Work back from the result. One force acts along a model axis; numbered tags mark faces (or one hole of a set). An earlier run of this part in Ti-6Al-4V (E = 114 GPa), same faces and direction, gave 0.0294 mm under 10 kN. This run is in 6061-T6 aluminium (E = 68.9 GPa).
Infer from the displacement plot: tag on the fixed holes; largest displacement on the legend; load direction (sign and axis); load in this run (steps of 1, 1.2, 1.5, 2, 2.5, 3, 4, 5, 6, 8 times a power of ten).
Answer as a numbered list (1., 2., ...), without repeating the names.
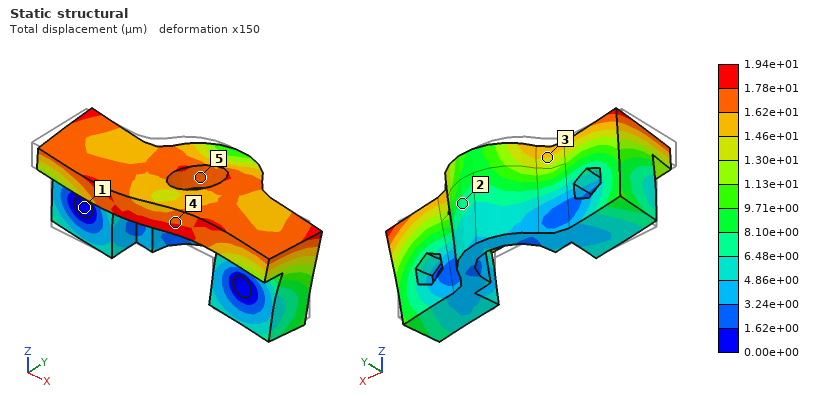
1. 1
2. 1.94e+01 µm
3. +X
4. 4 kN
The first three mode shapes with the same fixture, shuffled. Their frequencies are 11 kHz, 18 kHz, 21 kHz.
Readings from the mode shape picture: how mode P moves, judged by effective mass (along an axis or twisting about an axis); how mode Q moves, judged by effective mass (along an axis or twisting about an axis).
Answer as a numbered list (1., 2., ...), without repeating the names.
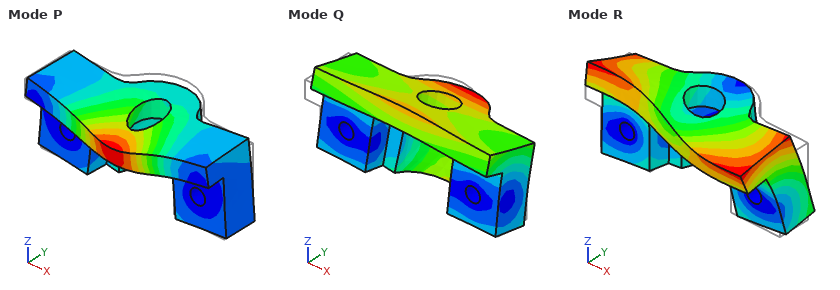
1. along Z
2. along Y
